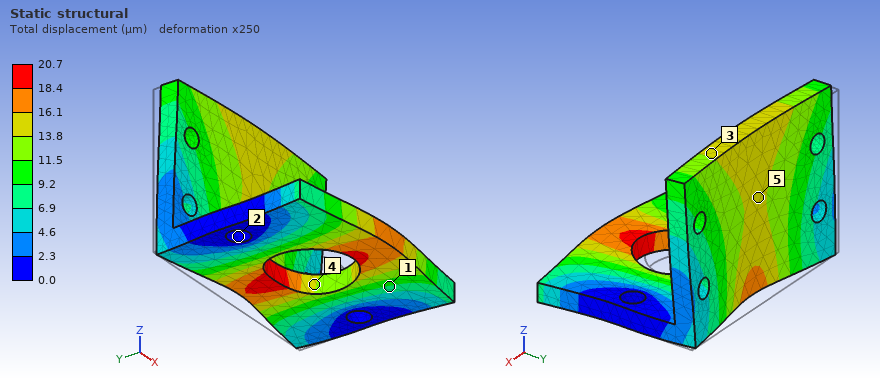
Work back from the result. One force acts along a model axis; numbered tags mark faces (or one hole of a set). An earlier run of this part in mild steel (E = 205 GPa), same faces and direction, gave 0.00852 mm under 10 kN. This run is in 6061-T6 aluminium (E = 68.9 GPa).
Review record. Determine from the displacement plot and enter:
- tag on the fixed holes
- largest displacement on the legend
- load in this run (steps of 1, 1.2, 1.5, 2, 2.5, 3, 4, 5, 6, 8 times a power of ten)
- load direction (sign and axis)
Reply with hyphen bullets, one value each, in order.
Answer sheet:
- 2
- 20.7 µm
- 8 kN
- -Y
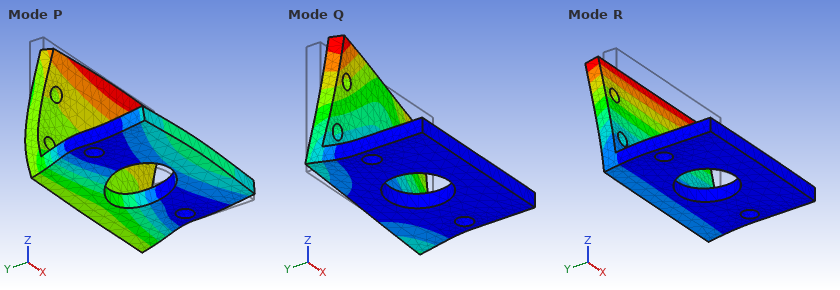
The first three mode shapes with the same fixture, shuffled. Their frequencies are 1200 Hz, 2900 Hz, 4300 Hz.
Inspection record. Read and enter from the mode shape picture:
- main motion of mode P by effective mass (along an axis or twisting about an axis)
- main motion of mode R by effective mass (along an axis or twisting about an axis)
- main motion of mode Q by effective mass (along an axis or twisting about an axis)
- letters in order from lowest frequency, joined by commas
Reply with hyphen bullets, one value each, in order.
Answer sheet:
- along Z
- along Y
- along X
- R, Q, P
